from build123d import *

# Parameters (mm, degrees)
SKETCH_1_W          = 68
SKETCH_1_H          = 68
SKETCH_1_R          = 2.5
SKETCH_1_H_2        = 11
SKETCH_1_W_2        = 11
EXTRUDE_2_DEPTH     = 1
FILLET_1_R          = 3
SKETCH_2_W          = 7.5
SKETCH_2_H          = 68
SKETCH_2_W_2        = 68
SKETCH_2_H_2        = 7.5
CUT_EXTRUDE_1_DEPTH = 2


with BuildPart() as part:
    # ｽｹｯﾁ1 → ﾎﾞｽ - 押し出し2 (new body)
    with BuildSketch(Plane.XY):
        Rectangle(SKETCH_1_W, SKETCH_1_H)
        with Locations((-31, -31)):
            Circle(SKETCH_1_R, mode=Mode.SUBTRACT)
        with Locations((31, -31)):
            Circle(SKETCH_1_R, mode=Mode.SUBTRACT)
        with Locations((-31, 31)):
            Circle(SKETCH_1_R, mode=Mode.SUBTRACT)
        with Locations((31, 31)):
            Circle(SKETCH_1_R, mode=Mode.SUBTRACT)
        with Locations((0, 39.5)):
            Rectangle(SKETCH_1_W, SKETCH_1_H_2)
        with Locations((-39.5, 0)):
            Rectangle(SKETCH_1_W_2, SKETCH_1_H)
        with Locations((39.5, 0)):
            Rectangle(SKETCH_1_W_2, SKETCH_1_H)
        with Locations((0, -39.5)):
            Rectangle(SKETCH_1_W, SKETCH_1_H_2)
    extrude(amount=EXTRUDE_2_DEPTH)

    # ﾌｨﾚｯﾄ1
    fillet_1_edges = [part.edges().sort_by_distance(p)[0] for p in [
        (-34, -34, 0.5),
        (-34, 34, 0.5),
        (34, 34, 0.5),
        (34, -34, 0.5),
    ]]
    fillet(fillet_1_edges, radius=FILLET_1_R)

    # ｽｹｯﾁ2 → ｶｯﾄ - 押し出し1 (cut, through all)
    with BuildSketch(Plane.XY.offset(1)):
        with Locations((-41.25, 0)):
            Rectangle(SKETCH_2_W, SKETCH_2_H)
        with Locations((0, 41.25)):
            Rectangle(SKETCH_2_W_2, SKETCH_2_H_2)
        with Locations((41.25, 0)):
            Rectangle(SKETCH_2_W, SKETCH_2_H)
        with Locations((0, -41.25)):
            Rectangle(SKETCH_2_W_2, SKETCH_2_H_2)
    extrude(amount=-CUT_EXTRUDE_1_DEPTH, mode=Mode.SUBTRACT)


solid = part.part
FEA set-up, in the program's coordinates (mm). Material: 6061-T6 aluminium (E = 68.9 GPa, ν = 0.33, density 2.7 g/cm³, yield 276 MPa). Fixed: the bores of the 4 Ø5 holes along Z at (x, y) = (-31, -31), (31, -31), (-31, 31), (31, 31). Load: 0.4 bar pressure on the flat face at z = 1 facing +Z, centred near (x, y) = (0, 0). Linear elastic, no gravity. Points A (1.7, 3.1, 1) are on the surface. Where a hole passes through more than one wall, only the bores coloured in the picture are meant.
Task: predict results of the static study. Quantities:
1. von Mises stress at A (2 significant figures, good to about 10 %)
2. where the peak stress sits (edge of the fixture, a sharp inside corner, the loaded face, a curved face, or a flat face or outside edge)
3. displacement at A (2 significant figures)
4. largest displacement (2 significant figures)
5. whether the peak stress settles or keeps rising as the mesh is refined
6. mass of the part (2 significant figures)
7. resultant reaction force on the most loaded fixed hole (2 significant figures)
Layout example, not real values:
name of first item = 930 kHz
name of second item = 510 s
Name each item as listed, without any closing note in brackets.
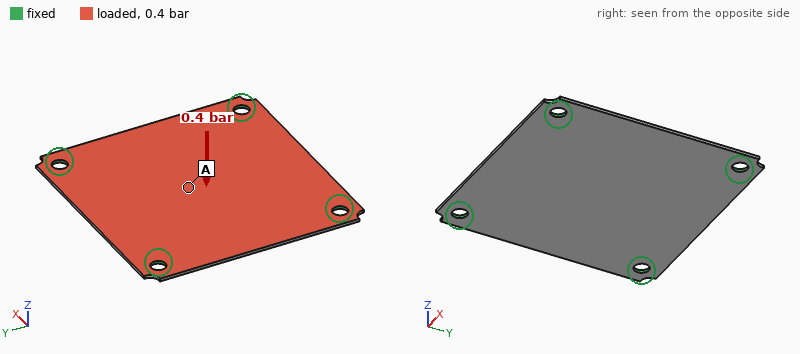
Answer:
von Mises stress at A = 45 MPa
where the peak stress sits = edge of the fixture
displacement at A = 0.57 mm
largest displacement = 0.58 mm
whether the peak stress settles or keeps rising as the mesh is refined = keeps rising
mass of the part = 15 g
resultant reaction force on the most loaded fixed hole = 55 N
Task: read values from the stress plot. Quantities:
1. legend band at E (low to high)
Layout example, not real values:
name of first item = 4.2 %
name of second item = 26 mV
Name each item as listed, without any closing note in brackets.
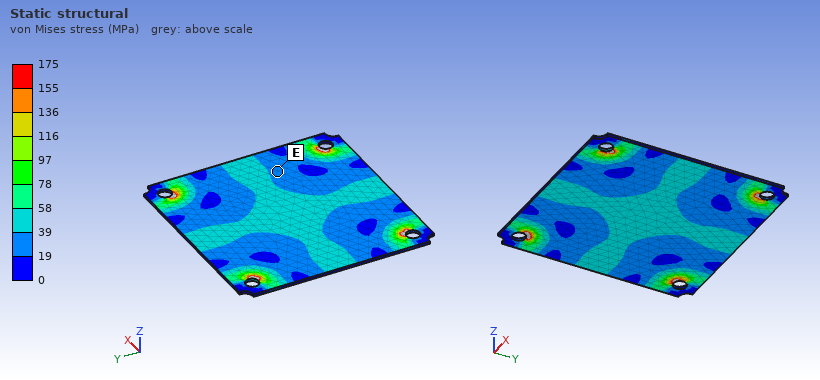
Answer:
legend band at E = 19 to 39 MPa
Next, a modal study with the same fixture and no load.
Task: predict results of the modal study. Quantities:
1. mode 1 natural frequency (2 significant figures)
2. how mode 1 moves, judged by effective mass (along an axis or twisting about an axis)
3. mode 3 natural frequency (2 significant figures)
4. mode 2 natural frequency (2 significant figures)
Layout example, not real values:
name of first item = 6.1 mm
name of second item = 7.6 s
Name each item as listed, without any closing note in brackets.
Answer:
mode 1 natural frequency = 990 Hz
how mode 1 moves, judged by effective mass = along Z
mode 3 natural frequency = 1700 Hz
mode 2 natural frequency = 1700 Hz
